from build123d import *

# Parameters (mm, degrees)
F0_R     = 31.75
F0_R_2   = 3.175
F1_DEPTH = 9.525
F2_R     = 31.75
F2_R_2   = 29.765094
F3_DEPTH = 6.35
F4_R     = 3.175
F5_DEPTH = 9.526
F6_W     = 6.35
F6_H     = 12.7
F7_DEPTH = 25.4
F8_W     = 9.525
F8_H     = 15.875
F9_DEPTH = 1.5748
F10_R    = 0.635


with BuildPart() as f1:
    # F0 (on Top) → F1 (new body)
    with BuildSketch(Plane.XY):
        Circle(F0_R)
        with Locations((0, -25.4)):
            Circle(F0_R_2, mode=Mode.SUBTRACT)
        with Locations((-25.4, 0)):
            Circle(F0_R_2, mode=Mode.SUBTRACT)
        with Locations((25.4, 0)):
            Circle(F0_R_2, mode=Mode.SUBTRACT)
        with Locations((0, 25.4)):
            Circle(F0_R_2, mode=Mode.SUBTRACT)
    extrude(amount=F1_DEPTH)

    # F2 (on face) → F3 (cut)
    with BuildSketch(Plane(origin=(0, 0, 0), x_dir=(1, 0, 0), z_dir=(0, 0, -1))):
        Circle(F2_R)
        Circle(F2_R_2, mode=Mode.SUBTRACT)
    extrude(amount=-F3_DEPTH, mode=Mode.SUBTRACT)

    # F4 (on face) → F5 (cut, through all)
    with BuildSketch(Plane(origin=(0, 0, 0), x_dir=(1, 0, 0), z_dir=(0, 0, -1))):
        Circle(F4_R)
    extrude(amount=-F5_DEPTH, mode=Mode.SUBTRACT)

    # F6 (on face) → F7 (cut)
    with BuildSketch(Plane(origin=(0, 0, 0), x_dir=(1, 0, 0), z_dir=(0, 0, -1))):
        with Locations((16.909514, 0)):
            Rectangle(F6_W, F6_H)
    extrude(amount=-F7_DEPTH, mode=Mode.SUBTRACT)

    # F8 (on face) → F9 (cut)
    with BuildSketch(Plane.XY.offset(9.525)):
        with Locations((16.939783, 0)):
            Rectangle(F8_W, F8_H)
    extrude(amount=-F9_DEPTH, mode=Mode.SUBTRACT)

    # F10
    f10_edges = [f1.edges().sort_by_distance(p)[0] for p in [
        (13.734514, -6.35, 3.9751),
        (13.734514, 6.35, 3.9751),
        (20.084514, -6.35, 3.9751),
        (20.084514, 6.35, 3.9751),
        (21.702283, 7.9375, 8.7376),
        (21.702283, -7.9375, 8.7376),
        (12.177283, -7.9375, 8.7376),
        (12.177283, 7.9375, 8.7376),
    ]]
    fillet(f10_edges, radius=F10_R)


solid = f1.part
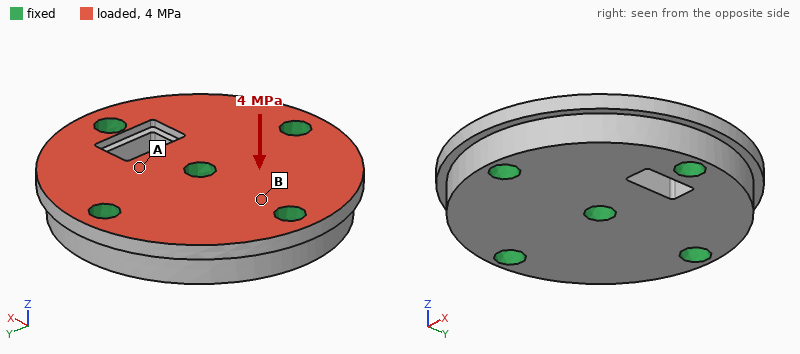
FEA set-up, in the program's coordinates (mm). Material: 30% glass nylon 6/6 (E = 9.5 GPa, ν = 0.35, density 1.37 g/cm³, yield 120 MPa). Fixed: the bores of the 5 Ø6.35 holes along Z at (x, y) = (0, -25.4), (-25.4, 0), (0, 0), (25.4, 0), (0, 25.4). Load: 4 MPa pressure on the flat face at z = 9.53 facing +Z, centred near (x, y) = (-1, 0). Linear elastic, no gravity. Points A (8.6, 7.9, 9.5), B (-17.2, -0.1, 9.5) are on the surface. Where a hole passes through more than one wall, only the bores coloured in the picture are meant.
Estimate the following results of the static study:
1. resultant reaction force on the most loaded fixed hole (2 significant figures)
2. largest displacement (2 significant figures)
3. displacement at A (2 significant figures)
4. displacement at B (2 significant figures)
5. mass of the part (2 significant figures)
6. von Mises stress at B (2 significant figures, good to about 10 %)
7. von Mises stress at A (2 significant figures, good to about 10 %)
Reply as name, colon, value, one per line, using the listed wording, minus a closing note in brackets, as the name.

resultant reaction force on the most loaded fixed hole: 2.4 kN
largest displacement: 90 µm
displacement at A: 25 µm
displacement at B: 16 µm
mass of the part: 35 g
von Mises stress at B: 17 MPa
von Mises stress at A: 5.0 MPa
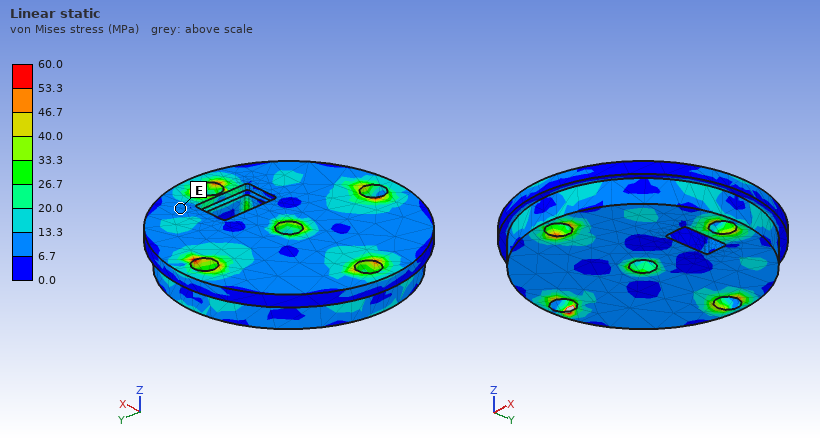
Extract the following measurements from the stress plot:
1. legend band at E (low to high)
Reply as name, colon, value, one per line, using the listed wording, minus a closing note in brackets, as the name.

legend band at E: 6.7 to 13.3 MPa
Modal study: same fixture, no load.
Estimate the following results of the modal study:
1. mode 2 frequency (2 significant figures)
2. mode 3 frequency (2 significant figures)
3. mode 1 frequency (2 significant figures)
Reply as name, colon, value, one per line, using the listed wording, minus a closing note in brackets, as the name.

mode 2 frequency: 14 kHz
mode 3 frequency: 14 kHz
mode 1 frequency: 13 kHz
